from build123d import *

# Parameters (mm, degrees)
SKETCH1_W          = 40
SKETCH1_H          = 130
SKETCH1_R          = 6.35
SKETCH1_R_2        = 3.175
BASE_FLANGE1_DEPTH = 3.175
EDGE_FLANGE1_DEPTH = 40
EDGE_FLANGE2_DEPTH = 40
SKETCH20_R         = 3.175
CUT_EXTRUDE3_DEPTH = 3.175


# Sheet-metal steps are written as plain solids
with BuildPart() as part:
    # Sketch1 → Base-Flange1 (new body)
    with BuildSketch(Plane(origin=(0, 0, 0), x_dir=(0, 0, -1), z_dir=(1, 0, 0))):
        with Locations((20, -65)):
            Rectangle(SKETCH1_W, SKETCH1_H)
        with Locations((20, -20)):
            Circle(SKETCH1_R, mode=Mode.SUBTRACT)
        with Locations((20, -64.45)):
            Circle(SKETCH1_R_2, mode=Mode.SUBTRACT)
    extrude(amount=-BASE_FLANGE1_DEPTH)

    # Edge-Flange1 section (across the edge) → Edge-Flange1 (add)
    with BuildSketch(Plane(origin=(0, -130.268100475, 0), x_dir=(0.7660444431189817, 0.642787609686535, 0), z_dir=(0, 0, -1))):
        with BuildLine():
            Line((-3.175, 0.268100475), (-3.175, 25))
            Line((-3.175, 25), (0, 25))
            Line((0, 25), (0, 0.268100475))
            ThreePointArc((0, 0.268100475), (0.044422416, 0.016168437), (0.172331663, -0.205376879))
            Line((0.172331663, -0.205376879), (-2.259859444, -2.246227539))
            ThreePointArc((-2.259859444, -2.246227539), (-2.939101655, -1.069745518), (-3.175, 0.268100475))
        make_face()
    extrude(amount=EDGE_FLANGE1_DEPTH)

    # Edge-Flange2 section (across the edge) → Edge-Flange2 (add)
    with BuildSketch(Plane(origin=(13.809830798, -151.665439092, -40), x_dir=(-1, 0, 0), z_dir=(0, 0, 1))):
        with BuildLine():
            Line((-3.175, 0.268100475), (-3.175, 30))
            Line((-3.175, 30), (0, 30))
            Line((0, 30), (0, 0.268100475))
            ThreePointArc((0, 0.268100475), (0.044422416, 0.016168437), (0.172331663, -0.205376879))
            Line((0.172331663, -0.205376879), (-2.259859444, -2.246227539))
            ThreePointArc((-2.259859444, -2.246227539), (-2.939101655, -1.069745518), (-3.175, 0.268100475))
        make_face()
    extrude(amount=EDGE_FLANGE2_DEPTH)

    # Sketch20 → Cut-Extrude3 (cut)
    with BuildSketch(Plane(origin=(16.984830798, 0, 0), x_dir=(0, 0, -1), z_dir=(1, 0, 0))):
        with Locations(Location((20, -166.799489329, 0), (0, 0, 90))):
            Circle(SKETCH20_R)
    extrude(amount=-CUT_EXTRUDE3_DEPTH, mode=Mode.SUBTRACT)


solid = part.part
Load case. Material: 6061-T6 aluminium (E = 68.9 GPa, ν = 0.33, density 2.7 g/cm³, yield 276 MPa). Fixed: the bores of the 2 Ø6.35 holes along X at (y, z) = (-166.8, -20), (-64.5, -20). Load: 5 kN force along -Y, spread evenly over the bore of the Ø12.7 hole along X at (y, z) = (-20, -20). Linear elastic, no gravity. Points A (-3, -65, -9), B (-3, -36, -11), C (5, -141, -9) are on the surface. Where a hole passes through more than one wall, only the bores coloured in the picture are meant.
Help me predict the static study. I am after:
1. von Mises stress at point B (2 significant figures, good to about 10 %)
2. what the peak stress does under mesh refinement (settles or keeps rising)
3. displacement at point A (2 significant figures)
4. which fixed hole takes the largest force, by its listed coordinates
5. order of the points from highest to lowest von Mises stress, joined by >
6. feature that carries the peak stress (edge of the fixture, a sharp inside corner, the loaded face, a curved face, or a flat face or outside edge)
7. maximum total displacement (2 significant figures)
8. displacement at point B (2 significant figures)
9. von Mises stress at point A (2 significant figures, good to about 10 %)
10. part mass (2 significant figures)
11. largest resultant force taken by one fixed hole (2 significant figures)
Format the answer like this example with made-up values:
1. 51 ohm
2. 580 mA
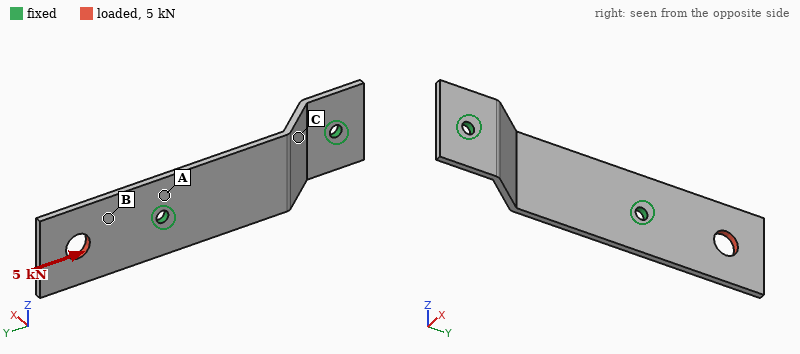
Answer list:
1. 45 MPa
2. keeps rising
3. 8.4 µm
4. (-64.5, -20)
5. B > A > C
6. edge of the fixture
7. 45 µm
8. 23 µm
9. 22 MPa
10. 63 g
11. 5.0 kN
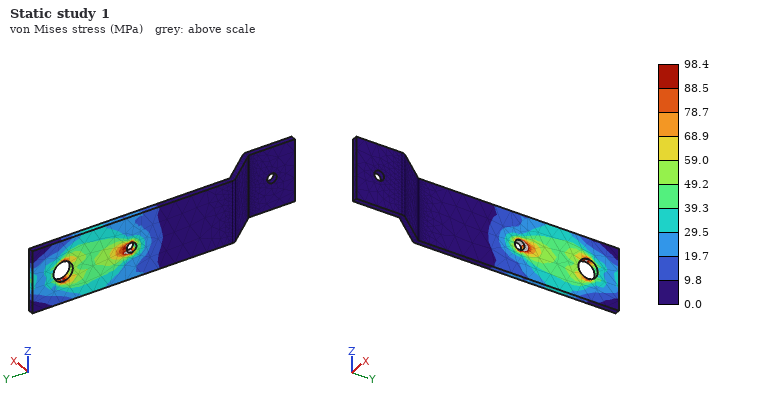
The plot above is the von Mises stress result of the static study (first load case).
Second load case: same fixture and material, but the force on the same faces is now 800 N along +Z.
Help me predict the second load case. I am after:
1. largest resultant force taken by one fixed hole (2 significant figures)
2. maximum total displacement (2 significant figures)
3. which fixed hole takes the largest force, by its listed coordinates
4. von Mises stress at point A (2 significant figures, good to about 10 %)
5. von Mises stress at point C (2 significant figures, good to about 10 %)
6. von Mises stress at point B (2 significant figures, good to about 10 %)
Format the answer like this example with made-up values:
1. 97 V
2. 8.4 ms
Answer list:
1. 1.0 kN
2. 0.16 mm
3. (-64.5, -20)
4. 22 MPa
5. 16 MPa
6. 13 MPa
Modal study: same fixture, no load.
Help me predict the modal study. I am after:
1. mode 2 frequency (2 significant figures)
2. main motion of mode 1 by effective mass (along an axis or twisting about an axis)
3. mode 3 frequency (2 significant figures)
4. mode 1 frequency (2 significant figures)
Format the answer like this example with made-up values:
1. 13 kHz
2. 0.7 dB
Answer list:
1. 1900 Hz
2. along X
3. 2200 Hz
4. 650 Hz
